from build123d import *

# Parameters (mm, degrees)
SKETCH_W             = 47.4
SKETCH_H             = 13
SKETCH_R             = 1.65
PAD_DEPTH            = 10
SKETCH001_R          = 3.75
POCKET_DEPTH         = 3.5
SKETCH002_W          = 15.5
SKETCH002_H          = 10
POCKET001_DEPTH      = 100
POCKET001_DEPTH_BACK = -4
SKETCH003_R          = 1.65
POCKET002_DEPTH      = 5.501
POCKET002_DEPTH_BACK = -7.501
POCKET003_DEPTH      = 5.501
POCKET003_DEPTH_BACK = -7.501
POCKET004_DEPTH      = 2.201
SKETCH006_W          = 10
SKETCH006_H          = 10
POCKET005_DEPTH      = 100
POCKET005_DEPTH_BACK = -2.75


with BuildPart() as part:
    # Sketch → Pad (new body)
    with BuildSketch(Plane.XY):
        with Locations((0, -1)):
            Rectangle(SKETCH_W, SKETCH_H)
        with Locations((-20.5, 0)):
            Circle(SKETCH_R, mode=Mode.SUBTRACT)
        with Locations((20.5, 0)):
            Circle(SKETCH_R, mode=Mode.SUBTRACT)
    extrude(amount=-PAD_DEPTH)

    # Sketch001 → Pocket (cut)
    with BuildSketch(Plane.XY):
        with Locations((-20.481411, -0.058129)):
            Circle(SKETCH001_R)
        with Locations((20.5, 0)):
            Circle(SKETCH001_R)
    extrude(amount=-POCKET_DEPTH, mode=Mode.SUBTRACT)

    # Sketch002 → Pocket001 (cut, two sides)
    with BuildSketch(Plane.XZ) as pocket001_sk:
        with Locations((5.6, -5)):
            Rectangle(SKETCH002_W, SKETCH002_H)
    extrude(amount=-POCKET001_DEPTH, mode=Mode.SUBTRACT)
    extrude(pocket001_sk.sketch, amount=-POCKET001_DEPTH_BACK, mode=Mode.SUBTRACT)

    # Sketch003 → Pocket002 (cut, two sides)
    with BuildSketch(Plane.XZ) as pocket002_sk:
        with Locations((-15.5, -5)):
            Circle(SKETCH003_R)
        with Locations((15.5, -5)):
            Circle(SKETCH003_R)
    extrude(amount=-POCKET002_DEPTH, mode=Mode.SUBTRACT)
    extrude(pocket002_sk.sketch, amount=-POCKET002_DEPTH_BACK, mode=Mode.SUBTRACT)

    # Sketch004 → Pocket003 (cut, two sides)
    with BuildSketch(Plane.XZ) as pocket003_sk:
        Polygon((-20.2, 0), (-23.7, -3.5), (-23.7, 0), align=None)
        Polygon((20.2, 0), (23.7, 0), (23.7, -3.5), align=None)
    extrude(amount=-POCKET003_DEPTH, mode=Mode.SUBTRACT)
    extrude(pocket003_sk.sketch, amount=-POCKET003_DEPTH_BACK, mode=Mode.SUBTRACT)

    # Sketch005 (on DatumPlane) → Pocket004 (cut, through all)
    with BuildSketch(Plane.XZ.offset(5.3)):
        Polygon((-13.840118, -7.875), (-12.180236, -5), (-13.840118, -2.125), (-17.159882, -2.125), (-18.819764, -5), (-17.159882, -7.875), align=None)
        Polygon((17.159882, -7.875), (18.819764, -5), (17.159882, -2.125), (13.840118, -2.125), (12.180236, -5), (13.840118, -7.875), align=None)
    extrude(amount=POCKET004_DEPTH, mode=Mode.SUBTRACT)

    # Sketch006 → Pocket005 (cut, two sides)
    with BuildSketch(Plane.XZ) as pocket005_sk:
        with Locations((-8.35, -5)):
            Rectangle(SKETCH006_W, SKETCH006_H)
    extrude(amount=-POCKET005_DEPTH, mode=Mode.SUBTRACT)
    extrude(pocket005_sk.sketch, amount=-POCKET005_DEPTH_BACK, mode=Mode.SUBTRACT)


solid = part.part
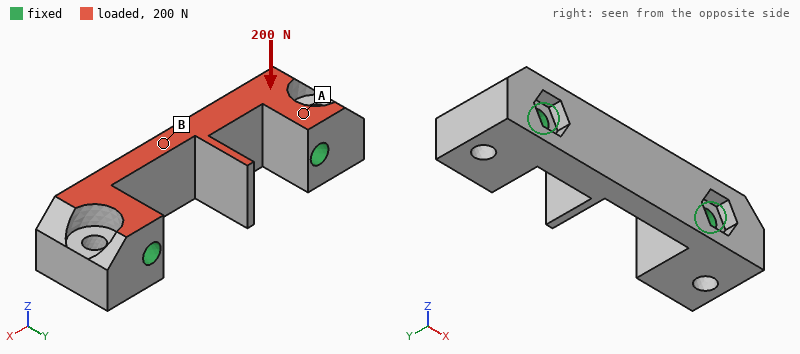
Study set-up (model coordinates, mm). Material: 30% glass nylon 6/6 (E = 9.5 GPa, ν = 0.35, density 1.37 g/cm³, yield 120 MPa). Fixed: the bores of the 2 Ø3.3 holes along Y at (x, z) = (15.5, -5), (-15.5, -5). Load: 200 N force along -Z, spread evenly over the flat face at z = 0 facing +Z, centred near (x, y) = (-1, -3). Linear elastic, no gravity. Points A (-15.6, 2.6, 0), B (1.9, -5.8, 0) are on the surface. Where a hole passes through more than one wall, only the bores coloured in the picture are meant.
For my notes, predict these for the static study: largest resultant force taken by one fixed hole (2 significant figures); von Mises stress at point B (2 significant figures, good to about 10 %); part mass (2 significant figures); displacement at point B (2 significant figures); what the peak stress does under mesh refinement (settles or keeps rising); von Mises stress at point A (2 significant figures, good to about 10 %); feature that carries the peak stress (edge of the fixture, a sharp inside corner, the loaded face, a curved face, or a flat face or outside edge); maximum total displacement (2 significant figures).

110 N
3.1 MPa
4.2 g
8.3 µm
keeps rising
0.94 MPa
edge of the fixture
14 µm
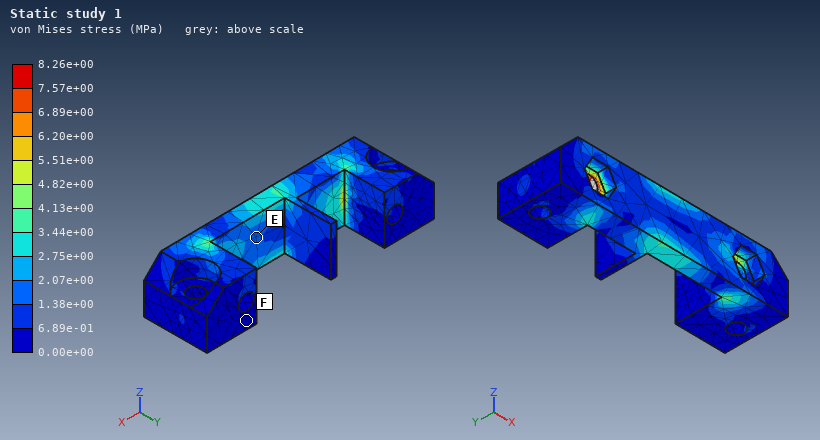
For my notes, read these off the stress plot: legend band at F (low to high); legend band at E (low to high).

0.00e+00 to 6.89e-01 MPa
1.38e+00 to 2.07e+00 MPa
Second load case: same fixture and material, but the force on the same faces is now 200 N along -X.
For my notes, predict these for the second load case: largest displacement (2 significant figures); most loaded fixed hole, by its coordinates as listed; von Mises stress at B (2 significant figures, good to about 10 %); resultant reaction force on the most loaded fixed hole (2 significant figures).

81 µm
(-15.5, -5)
1.4 MPa
110 N
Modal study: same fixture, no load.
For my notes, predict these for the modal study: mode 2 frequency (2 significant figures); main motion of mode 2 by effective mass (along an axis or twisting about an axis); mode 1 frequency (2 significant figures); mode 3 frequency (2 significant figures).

9400 Hz
along Y
6700 Hz
12 kHz
